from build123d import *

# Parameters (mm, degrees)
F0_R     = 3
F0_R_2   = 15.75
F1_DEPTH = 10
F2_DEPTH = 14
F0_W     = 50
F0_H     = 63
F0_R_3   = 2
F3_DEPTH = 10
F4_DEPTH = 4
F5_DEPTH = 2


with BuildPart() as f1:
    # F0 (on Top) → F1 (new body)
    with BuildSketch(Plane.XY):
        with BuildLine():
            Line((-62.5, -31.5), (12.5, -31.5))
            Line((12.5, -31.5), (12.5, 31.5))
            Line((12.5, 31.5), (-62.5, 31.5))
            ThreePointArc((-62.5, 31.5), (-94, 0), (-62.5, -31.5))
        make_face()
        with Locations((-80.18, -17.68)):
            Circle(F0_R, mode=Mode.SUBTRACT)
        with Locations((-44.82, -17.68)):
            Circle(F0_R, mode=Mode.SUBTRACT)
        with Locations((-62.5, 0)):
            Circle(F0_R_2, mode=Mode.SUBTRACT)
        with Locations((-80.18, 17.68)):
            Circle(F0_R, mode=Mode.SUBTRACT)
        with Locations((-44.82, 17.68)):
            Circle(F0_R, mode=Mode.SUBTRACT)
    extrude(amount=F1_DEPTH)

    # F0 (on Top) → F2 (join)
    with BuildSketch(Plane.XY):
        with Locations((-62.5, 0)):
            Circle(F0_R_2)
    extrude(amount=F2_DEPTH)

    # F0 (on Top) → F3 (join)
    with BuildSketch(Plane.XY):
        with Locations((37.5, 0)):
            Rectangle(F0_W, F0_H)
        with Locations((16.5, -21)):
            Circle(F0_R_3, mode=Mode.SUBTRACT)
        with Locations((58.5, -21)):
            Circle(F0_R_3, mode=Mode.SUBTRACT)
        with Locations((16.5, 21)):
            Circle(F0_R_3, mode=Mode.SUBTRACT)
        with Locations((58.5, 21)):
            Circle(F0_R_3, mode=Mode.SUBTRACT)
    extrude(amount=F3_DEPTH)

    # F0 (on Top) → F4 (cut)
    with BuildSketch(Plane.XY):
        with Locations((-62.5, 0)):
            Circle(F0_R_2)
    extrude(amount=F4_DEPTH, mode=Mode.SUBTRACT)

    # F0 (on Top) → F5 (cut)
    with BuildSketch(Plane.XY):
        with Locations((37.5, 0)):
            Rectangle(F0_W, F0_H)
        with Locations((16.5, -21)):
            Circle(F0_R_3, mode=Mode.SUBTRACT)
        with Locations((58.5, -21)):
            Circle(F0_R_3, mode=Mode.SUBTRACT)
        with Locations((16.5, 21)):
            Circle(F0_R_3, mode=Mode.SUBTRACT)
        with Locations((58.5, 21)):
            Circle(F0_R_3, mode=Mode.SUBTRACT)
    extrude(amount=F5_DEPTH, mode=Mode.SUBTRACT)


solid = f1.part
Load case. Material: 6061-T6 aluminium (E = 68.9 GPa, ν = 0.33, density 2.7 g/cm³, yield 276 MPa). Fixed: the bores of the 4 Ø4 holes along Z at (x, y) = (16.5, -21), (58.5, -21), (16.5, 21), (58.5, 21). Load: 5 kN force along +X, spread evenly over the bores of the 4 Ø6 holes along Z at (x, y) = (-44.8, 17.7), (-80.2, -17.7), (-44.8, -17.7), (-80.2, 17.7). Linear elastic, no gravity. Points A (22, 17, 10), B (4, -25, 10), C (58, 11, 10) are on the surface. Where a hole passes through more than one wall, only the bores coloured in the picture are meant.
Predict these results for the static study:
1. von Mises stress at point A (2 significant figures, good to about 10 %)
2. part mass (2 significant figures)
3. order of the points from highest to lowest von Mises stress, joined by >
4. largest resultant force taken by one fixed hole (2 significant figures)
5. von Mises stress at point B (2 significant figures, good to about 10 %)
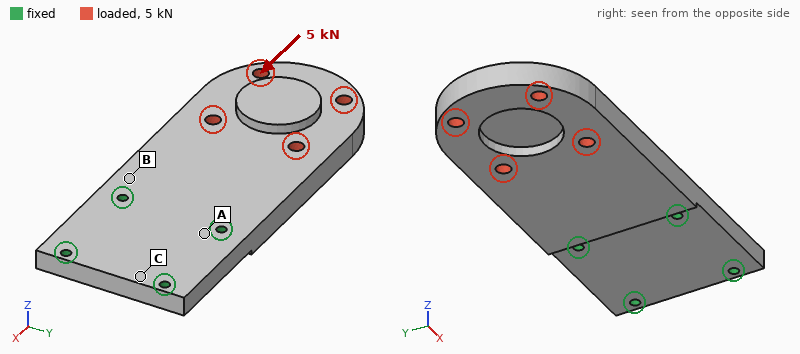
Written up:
6.0 MPa
230 g
B > A > C
2.1 kN
9.5 MPa
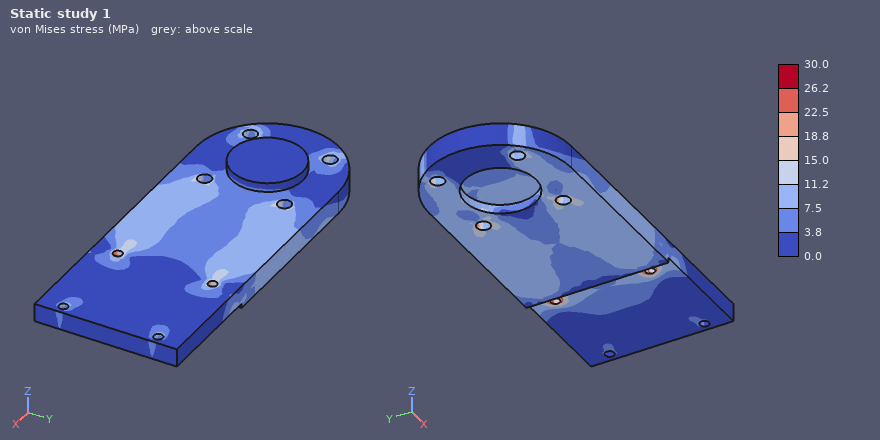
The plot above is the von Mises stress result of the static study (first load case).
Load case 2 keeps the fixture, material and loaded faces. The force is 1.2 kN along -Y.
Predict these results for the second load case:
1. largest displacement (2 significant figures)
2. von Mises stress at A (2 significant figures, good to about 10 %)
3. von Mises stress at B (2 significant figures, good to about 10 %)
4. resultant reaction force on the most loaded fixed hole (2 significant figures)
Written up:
37 µm
3.5 MPa
12 MPa
2.0 kN
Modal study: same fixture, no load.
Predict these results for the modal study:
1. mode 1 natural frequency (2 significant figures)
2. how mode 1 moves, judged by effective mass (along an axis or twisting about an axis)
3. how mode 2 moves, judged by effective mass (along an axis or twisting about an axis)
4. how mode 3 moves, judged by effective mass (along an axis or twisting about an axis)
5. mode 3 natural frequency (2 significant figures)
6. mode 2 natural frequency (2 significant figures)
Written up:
640 Hz
along Z
twisting about X
along Y
3500 Hz
2600 Hz
